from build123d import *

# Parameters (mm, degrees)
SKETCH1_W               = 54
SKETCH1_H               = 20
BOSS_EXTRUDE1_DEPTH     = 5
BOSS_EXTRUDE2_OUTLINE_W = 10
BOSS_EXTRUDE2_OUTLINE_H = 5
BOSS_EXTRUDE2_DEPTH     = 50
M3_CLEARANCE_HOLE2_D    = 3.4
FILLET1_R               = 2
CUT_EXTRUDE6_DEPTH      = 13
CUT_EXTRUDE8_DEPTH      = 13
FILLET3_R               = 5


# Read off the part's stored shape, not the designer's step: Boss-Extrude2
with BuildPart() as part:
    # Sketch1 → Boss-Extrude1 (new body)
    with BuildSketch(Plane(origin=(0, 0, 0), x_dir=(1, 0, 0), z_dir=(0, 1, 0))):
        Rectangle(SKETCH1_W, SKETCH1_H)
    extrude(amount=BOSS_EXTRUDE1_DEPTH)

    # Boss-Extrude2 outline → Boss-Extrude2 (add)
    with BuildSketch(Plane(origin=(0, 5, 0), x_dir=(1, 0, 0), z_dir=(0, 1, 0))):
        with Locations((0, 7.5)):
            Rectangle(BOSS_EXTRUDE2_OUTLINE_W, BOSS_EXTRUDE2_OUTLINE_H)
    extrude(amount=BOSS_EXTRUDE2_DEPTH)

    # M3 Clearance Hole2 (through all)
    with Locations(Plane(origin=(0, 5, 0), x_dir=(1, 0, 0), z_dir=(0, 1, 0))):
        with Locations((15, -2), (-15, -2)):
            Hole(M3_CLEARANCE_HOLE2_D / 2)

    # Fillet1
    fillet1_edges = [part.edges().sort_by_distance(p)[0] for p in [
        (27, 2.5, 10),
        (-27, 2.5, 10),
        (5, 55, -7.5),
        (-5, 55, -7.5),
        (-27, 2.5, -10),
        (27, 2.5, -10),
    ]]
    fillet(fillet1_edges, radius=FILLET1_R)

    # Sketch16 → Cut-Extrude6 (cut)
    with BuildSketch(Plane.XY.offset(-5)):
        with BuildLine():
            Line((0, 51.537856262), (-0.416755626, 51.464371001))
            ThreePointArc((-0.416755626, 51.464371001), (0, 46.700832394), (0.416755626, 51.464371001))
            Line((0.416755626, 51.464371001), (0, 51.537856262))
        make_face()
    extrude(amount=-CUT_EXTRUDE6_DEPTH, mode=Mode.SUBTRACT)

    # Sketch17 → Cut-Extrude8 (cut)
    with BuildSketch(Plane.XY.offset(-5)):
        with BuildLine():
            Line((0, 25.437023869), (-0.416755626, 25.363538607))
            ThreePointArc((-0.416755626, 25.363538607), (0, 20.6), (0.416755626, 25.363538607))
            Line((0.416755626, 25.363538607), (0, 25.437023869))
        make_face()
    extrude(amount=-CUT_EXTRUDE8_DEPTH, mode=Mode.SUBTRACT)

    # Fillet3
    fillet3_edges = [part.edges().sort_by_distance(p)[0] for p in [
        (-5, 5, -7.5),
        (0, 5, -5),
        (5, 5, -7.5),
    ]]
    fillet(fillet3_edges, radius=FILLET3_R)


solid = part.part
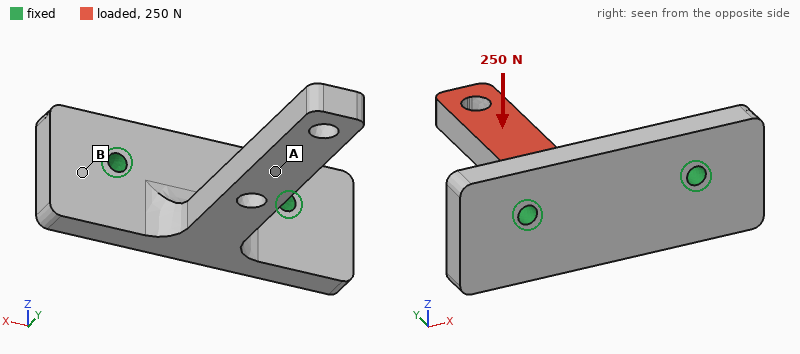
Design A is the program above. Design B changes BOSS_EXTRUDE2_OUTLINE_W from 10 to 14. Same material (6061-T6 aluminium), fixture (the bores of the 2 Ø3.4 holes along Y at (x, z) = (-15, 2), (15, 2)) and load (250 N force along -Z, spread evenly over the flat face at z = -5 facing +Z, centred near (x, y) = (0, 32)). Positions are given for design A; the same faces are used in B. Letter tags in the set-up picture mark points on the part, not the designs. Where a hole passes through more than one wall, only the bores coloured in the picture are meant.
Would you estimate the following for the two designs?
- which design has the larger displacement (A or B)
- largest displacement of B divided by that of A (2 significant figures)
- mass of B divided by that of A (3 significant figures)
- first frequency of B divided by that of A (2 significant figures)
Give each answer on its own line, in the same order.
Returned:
A
0.73
1.13
0.97
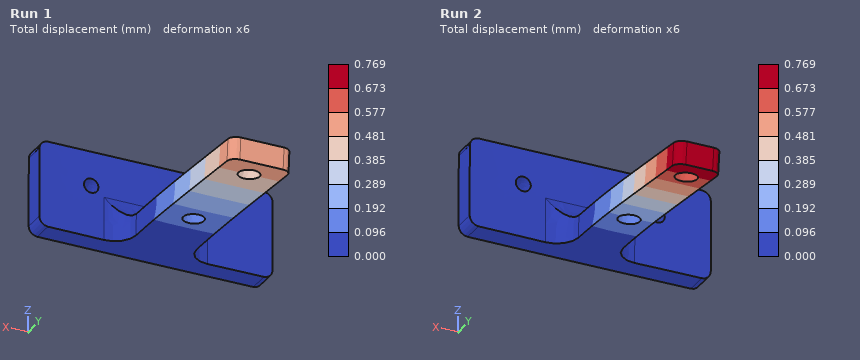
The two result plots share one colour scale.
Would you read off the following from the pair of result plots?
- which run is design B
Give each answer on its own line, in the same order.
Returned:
Run 1
